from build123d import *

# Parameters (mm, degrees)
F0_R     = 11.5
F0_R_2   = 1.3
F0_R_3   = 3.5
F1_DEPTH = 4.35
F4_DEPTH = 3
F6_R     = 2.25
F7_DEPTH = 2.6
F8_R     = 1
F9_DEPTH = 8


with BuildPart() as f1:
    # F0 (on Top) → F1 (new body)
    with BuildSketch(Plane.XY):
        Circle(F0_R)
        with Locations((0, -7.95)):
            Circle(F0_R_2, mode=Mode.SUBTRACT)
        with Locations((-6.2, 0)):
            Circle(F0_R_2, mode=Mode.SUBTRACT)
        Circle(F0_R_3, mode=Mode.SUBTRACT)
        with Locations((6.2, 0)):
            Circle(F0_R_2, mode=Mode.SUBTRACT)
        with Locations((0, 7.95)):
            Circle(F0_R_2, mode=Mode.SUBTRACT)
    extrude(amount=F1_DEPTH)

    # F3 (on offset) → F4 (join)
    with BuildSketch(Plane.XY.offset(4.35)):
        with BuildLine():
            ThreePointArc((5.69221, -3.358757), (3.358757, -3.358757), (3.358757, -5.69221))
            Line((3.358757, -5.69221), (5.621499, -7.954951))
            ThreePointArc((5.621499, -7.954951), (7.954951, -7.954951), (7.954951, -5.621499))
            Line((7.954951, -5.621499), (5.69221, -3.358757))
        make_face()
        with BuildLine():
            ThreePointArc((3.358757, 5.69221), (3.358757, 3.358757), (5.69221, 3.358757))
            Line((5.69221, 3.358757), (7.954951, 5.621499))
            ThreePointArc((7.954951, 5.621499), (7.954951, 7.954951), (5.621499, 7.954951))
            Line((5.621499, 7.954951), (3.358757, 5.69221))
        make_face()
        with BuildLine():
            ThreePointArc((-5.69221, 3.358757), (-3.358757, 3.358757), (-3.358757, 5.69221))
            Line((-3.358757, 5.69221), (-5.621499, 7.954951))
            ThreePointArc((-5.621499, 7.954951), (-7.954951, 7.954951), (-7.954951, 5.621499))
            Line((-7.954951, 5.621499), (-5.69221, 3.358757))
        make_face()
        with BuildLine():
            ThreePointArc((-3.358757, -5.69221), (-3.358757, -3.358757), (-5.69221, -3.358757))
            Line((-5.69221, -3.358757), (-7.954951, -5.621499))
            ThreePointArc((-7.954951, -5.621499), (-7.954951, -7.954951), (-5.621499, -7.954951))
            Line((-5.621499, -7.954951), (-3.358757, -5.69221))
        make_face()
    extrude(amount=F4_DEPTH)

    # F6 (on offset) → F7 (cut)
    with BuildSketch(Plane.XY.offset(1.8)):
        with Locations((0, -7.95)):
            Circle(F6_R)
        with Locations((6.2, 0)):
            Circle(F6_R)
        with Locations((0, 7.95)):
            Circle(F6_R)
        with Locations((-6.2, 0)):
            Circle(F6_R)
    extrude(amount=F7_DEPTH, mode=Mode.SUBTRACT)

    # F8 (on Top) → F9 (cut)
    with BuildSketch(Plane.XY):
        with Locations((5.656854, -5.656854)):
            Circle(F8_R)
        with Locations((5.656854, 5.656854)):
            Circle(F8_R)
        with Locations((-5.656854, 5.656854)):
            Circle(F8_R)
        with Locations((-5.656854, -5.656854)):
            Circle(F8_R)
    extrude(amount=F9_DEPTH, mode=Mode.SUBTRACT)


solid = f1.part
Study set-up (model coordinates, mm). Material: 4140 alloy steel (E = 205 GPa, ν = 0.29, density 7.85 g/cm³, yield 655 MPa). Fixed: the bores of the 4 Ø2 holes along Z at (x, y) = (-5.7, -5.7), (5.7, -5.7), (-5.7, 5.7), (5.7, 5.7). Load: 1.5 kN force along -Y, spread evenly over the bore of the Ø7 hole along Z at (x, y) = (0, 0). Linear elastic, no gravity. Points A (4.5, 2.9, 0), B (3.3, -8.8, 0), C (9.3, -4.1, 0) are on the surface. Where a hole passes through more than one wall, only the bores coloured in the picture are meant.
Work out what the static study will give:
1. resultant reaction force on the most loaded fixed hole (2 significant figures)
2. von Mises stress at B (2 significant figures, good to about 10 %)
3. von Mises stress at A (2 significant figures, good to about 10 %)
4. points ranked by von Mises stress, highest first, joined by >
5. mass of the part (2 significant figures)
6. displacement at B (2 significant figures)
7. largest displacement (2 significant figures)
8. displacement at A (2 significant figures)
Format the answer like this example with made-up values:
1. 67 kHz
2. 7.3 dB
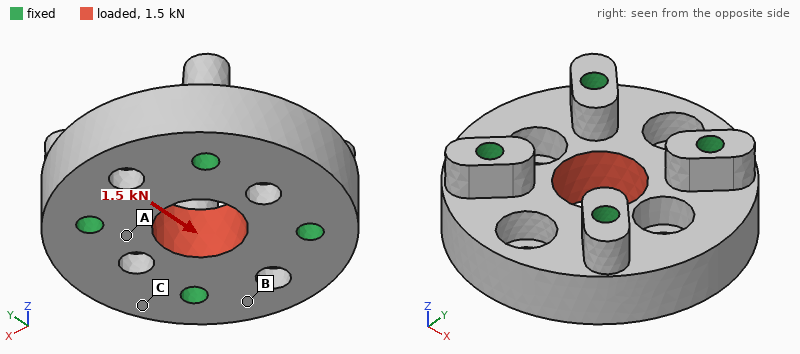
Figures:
1. 390 N
2. 12 MPa
3. 18 MPa
4. A > B > C
5. 12 g
6. 0.33 µm
7. 0.86 µm
8. 0.26 µm
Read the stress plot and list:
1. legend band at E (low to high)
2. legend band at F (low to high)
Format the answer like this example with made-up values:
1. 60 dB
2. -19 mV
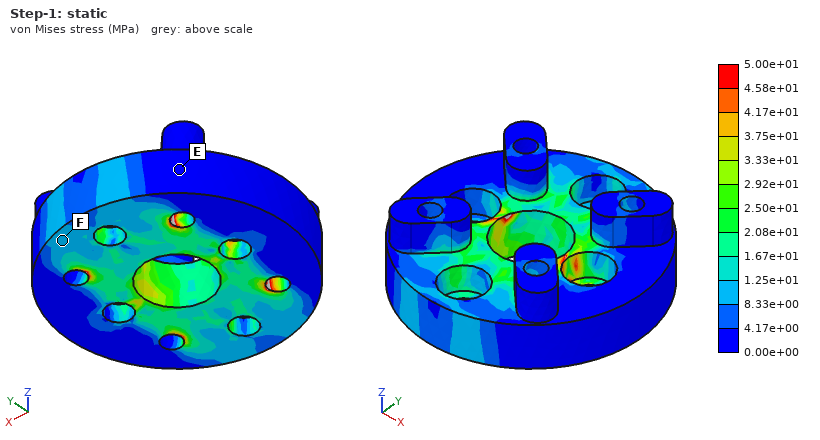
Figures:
1. 0.00e+00 to 4.17e+00 MPa
2. 8.33e+00 to 1.25e+01 MPa
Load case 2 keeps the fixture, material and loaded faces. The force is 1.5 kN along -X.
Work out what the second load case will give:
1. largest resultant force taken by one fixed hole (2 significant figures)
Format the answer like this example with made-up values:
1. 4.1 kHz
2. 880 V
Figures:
1. 390 N
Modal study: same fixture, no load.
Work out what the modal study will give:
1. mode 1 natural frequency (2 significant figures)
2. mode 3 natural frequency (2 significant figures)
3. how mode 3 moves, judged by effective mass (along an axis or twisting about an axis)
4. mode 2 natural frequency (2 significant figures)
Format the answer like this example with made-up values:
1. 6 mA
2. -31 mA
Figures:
1. 79 kHz
2. 85 kHz
3. twisting about X
4. 81 kHz
